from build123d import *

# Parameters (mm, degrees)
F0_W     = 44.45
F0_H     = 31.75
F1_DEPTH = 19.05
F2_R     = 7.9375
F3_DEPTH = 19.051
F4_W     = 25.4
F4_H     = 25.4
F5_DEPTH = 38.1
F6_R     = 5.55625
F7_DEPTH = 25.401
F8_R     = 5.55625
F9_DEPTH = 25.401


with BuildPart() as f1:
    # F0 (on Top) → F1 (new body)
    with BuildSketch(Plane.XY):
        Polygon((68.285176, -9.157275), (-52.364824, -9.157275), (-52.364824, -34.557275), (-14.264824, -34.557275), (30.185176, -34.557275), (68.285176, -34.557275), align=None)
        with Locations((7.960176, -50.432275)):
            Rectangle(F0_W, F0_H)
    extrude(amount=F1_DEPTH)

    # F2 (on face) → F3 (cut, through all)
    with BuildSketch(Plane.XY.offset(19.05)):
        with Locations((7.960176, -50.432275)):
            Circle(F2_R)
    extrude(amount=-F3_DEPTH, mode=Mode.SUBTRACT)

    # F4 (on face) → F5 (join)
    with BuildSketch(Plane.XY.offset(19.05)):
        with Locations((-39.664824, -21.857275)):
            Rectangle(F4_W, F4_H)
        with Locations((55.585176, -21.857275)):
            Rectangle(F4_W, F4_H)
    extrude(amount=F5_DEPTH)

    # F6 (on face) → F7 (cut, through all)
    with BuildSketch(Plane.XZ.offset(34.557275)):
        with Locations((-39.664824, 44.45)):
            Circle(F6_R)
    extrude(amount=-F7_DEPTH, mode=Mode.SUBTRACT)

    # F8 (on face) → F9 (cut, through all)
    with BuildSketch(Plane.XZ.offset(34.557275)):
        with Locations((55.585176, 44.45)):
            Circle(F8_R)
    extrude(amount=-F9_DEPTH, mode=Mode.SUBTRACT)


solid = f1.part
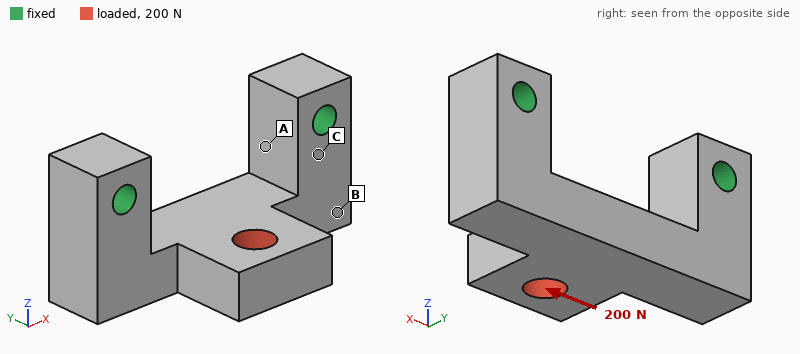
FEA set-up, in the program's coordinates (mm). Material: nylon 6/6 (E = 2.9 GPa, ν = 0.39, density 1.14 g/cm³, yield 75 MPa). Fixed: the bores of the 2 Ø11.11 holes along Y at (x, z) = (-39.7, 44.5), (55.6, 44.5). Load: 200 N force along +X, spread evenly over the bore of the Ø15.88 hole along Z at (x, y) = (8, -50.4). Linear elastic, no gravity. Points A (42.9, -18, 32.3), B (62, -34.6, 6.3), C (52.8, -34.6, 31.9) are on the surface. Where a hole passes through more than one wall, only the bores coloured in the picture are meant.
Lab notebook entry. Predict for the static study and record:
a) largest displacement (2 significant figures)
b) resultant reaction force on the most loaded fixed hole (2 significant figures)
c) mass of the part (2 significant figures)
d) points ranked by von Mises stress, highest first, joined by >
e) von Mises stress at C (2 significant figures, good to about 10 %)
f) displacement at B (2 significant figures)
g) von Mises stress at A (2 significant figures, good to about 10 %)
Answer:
48 µm
120 N
140 g
C > A > B
0.57 MPa
17 µm
0.36 MPa
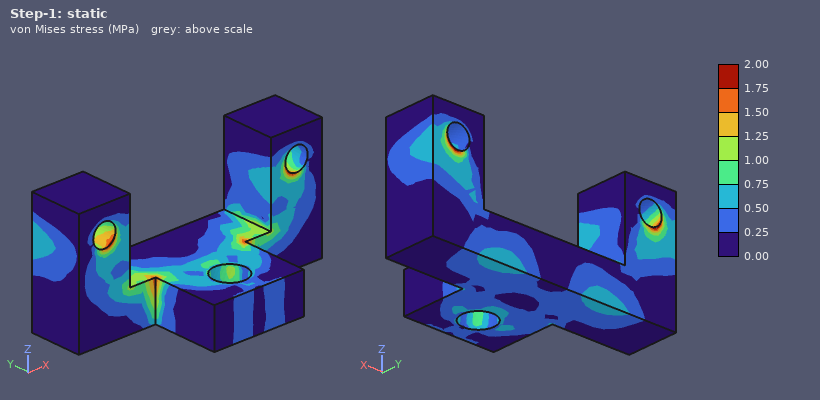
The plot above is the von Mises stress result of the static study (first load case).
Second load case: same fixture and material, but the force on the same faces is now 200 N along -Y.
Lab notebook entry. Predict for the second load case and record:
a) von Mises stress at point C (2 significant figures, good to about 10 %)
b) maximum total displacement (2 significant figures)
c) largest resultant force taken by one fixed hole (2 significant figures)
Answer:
1.2 MPa
50 µm
100 N
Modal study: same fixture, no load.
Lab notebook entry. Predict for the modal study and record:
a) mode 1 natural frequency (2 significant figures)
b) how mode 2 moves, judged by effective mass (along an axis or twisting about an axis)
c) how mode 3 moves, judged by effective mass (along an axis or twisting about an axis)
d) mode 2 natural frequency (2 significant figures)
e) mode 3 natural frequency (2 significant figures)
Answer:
1100 Hz
along Y
along X
1600 Hz
1700 Hz
